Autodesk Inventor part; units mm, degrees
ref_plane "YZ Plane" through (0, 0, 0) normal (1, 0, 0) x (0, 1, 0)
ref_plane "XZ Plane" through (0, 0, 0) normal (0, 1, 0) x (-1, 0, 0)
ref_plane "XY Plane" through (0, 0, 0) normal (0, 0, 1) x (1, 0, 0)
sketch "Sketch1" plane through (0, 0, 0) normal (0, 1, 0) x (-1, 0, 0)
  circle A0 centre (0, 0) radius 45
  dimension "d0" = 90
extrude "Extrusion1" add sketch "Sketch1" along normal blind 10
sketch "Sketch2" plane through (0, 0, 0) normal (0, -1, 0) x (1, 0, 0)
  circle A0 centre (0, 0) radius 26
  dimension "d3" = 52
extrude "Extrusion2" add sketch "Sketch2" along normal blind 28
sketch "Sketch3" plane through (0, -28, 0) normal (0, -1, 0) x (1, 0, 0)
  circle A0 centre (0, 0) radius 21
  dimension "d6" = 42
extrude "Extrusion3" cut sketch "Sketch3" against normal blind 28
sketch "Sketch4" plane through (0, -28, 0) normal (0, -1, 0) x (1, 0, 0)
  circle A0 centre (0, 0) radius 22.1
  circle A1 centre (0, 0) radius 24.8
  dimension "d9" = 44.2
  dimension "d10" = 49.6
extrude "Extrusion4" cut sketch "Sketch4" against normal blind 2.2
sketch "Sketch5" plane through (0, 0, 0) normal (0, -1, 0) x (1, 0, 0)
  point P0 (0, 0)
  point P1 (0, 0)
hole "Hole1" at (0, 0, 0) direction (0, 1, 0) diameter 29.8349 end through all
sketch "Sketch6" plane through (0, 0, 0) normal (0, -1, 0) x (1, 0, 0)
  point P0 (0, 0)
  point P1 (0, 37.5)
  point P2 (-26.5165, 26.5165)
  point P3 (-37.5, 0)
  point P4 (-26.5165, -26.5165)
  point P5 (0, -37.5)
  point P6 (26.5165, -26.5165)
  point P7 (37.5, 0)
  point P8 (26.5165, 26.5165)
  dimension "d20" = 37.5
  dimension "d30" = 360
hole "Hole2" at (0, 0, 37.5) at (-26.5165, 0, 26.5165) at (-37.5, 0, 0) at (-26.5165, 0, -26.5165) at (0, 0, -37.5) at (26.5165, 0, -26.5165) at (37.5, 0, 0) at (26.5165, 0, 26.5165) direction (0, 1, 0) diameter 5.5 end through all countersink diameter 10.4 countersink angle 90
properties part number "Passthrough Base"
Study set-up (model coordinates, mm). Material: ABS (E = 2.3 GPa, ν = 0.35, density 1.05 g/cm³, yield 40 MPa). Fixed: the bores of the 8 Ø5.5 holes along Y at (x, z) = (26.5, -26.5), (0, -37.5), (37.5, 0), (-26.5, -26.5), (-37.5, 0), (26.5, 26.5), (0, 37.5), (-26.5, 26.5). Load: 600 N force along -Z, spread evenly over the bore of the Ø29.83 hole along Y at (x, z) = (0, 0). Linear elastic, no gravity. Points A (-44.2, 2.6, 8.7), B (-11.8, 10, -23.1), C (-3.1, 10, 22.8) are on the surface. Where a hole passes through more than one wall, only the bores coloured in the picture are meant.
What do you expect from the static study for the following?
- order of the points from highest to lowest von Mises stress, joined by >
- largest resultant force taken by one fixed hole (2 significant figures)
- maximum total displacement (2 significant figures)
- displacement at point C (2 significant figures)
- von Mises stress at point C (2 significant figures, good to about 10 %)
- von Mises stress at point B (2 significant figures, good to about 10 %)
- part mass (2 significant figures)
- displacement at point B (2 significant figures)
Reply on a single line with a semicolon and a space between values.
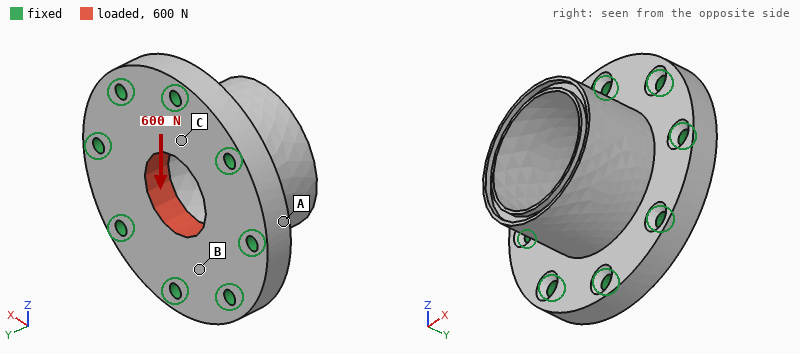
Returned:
C > B > A; 120 N; 7.3 µm; 4.7 µm; 0.69 MPa; 0.42 MPa; 78 g; 4.1 µm
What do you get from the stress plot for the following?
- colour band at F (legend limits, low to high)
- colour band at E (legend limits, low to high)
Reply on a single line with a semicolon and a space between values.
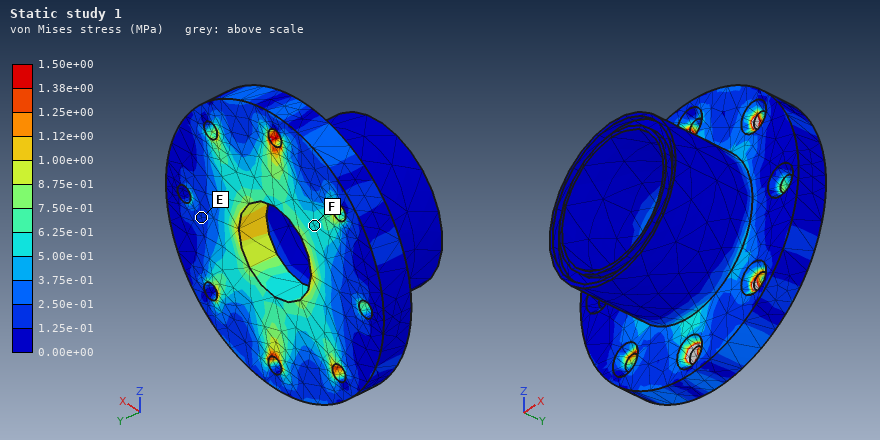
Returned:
5.00e-01 to 6.25e-01 MPa; 1.25e-01 to 2.50e-01 MPa
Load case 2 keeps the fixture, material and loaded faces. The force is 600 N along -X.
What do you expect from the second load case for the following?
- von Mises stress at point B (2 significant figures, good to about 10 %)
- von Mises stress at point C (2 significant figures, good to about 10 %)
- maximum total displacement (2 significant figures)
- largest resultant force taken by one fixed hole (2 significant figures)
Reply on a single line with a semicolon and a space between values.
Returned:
0.44 MPa; 0.38 MPa; 7.3 µm; 120 N
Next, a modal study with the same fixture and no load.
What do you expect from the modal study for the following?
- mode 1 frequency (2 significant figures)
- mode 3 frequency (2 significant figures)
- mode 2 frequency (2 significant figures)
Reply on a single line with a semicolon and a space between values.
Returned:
3500 Hz; 4000 Hz; 3500 Hz
